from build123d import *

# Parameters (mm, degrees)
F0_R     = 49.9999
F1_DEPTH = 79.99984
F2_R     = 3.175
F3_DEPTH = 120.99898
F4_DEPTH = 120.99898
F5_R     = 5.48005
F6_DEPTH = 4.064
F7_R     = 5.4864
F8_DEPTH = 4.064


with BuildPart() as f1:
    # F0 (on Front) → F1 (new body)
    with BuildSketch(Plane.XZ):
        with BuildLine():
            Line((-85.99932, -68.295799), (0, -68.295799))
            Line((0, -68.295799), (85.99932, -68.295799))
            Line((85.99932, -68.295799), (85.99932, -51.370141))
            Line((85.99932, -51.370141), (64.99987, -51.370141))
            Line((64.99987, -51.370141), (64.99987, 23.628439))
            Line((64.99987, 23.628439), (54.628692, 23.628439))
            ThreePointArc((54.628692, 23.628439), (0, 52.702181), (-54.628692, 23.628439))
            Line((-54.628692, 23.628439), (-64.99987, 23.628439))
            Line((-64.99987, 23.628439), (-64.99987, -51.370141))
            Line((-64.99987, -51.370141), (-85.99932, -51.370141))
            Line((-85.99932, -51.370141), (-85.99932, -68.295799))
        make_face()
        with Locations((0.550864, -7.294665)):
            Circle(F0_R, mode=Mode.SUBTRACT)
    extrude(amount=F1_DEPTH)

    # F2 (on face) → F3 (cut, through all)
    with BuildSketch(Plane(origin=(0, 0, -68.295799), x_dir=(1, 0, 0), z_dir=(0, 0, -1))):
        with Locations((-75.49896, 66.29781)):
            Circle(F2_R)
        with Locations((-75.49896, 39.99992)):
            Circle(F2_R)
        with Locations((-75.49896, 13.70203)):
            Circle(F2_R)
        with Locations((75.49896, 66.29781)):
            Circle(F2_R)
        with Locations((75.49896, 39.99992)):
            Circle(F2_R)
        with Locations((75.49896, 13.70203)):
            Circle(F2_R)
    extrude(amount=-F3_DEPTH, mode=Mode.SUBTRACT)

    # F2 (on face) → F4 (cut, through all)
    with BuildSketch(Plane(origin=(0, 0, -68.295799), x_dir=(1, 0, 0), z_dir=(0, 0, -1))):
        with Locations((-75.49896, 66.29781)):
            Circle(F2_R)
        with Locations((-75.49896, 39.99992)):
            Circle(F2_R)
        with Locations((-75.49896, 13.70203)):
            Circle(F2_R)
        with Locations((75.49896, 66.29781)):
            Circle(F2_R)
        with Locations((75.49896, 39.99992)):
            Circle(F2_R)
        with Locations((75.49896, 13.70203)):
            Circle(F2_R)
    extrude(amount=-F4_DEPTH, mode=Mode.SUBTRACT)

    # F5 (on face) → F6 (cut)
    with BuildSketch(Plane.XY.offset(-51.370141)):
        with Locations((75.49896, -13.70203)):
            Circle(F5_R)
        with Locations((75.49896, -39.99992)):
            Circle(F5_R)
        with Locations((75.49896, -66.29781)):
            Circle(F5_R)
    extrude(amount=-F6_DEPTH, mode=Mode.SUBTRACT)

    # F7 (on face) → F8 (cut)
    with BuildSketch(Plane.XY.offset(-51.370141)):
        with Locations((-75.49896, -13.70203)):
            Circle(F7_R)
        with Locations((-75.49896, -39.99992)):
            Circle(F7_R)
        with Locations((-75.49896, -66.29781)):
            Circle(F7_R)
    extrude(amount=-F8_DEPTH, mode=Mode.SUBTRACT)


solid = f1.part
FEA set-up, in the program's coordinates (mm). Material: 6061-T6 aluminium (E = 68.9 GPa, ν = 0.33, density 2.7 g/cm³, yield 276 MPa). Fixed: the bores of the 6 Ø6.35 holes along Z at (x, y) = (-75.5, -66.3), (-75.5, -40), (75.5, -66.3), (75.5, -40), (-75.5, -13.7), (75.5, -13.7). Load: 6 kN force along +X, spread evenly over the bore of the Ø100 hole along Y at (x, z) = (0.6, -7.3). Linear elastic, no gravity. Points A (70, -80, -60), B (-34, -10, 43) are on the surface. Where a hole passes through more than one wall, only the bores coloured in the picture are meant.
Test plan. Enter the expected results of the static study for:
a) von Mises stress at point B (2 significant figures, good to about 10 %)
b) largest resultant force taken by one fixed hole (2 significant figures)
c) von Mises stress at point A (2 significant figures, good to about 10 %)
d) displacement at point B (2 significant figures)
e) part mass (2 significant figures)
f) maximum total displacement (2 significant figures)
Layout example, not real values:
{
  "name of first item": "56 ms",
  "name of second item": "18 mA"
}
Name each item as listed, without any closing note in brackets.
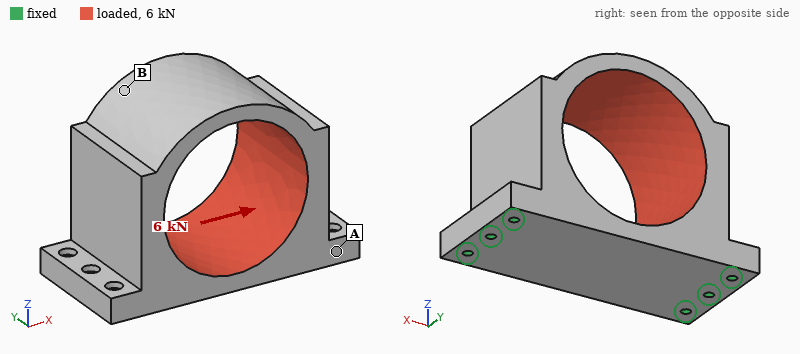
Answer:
{
  "von Mises stress at point B": "9.4 MPa",
  "largest resultant force taken by one fixed hole": "1.3 kN",
  "von Mises stress at point A": "2.2 MPa",
  "displacement at point B": "54 µm",
  "part mass": "1.5 kg",
  "maximum total displacement": "55 µm"
}
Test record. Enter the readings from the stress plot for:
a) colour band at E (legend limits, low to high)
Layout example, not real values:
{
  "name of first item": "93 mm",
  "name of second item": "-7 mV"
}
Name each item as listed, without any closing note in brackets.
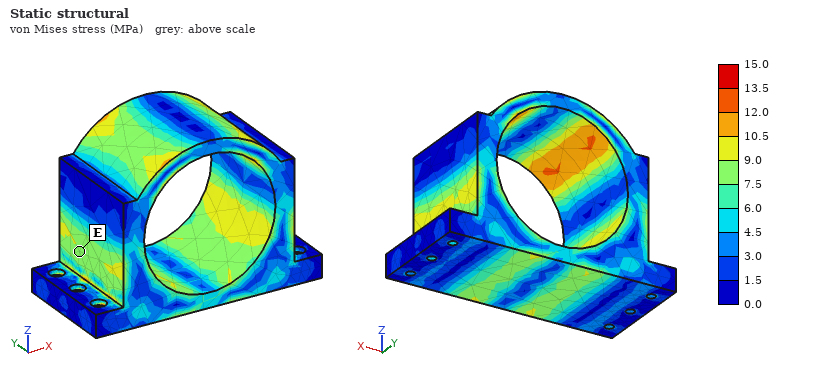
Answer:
{
  "colour band at E": "7.5 to 9.0 MPa"
}
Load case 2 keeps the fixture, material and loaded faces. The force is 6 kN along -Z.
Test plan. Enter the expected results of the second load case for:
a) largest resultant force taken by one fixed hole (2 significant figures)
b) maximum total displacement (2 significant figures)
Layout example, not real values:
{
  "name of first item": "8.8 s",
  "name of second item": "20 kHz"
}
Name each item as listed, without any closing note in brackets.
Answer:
{
  "largest resultant force taken by one fixed hole": "1.0 kN",
  "maximum total displacement": "14 µm"
}
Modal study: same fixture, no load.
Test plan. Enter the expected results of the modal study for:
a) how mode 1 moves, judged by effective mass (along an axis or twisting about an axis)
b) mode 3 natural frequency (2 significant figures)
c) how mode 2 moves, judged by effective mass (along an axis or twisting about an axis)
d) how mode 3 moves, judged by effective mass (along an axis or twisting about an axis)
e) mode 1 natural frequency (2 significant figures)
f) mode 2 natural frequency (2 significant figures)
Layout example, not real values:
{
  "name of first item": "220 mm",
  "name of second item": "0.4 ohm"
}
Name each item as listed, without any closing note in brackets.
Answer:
{
  "how mode 1 moves, judged by effective mass": "along X",
  "mode 3 natural frequency": "2800 Hz",
  "how mode 2 moves, judged by effective mass": "along Y",
  "how mode 3 moves, judged by effective mass": "along Z",
  "mode 1 natural frequency": "1900 Hz",
  "mode 2 natural frequency": "2000 Hz"
}
